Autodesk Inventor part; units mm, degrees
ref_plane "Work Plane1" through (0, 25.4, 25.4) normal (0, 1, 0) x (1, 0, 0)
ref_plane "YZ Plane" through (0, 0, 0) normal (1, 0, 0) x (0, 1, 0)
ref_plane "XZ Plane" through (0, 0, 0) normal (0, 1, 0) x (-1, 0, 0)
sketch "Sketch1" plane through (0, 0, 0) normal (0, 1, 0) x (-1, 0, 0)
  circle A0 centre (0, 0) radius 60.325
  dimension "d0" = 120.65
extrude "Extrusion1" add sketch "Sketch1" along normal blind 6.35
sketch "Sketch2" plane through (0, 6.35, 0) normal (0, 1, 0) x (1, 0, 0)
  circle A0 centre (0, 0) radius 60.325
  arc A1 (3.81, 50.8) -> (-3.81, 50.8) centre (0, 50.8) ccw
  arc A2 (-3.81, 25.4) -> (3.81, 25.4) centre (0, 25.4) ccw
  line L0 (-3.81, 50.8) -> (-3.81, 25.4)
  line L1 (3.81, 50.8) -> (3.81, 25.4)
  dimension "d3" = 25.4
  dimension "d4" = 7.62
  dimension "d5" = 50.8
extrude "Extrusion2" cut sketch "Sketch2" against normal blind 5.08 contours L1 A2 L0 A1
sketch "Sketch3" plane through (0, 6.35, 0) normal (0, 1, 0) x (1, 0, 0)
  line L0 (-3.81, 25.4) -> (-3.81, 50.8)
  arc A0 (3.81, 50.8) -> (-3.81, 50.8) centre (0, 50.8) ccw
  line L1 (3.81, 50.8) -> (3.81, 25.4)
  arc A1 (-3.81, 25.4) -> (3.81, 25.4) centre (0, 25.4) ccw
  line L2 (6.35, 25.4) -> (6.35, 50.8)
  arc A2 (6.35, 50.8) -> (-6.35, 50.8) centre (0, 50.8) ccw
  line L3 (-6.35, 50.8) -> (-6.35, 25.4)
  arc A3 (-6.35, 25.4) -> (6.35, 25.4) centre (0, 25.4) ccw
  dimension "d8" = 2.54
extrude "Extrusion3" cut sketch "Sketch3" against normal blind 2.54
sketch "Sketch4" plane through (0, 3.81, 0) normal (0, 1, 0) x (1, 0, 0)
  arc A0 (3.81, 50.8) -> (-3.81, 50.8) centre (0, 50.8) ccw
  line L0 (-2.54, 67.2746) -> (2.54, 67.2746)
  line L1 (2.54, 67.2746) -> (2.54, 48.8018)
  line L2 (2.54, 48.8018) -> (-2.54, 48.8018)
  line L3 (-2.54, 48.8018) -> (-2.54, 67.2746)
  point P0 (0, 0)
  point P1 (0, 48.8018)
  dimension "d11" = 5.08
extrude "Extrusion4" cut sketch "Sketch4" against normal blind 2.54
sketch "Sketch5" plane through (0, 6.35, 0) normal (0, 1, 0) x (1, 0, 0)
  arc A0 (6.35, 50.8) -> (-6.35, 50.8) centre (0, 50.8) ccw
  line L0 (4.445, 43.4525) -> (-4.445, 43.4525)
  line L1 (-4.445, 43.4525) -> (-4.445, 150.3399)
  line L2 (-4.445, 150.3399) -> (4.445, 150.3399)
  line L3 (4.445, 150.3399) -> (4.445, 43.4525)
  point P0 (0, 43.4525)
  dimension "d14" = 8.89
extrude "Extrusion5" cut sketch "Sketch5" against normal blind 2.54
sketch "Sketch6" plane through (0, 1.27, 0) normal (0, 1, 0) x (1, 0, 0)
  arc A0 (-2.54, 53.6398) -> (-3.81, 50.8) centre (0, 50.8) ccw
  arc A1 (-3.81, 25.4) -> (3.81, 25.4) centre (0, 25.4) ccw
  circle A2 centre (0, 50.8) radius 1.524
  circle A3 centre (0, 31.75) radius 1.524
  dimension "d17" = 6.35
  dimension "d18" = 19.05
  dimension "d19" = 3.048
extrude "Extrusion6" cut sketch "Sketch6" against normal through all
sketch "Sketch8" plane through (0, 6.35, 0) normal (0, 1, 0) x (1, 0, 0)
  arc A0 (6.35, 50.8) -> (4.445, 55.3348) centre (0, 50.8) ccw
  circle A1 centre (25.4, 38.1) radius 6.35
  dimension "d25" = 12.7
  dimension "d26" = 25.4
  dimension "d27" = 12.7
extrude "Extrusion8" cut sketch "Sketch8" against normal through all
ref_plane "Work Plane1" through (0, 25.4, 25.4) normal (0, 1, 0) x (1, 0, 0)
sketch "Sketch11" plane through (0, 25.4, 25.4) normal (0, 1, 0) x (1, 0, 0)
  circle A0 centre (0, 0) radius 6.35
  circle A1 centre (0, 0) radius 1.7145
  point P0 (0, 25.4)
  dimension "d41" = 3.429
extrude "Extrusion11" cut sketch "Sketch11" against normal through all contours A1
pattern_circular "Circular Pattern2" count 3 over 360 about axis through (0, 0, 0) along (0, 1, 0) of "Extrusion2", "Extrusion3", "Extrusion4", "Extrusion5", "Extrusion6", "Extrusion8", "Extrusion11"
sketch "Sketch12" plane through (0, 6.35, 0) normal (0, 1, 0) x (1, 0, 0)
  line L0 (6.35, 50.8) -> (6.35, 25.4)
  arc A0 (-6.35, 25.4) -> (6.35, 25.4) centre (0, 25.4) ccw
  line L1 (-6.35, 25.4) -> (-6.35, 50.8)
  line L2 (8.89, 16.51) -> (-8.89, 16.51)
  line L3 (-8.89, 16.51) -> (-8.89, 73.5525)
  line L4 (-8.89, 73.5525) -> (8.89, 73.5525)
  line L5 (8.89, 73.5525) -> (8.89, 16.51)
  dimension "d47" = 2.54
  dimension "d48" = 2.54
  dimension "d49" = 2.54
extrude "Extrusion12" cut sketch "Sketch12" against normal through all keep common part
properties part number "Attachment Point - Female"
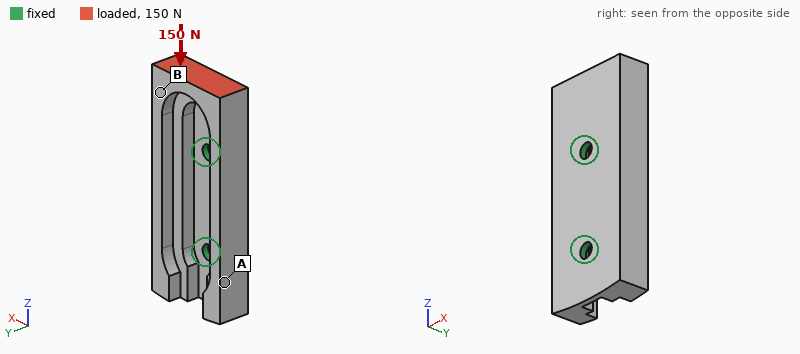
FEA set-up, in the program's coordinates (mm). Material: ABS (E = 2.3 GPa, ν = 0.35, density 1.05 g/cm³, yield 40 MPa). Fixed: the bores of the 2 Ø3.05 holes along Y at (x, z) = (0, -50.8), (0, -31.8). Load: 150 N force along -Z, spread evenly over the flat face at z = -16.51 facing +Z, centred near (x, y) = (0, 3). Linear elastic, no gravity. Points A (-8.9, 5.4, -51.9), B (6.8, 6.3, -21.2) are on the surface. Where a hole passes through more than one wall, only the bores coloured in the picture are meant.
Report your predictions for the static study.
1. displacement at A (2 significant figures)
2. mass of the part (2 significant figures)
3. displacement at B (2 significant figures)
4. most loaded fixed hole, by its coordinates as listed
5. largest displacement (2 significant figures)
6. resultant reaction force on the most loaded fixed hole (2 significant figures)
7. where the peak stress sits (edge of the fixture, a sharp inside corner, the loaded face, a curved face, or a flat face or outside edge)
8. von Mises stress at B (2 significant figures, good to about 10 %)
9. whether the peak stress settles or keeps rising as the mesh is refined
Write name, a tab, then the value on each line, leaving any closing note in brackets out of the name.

displacement at A	0.053 mm
mass of the part	3.1 g
displacement at B	0.11 mm
most loaded fixed hole, by its coordinates as listed	(0, -31.8)
largest displacement	0.16 mm
resultant reaction force on the most loaded fixed hole	90 N
where the peak stress sits	edge of the fixture
von Mises stress at B	3.6 MPa
whether the peak stress settles or keeps rising as the mesh is refined	keeps rising
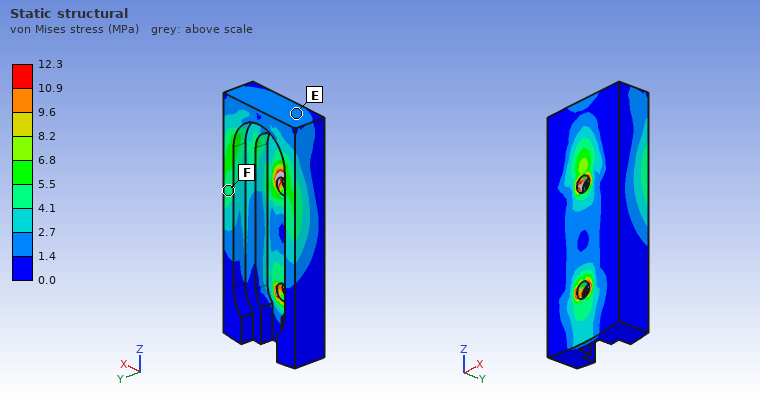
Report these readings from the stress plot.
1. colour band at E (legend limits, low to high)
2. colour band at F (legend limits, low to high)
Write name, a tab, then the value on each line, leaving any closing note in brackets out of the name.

colour band at E	1.4 to 2.7 MPa
colour band at F	4.1 to 5.5 MPa
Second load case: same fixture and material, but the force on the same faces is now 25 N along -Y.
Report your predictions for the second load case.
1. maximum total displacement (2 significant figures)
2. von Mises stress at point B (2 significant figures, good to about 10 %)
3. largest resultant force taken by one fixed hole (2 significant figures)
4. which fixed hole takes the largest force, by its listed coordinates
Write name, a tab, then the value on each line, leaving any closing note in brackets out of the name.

maximum total displacement	0.23 mm
von Mises stress at point B	2.1 MPa
largest resultant force taken by one fixed hole	49 N
which fixed hole takes the largest force, by its listed coordinates	(0, -31.8)
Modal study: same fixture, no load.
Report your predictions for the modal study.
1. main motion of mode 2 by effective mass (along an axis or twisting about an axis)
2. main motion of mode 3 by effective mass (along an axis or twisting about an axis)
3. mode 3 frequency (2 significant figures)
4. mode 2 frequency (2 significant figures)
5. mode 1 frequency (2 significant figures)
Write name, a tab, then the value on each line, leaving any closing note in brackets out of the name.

main motion of mode 2 by effective mass	along Y
main motion of mode 3 by effective mass	along Y
mode 3 frequency	2500 Hz
mode 2 frequency	2200 Hz
mode 1 frequency	1500 Hz
